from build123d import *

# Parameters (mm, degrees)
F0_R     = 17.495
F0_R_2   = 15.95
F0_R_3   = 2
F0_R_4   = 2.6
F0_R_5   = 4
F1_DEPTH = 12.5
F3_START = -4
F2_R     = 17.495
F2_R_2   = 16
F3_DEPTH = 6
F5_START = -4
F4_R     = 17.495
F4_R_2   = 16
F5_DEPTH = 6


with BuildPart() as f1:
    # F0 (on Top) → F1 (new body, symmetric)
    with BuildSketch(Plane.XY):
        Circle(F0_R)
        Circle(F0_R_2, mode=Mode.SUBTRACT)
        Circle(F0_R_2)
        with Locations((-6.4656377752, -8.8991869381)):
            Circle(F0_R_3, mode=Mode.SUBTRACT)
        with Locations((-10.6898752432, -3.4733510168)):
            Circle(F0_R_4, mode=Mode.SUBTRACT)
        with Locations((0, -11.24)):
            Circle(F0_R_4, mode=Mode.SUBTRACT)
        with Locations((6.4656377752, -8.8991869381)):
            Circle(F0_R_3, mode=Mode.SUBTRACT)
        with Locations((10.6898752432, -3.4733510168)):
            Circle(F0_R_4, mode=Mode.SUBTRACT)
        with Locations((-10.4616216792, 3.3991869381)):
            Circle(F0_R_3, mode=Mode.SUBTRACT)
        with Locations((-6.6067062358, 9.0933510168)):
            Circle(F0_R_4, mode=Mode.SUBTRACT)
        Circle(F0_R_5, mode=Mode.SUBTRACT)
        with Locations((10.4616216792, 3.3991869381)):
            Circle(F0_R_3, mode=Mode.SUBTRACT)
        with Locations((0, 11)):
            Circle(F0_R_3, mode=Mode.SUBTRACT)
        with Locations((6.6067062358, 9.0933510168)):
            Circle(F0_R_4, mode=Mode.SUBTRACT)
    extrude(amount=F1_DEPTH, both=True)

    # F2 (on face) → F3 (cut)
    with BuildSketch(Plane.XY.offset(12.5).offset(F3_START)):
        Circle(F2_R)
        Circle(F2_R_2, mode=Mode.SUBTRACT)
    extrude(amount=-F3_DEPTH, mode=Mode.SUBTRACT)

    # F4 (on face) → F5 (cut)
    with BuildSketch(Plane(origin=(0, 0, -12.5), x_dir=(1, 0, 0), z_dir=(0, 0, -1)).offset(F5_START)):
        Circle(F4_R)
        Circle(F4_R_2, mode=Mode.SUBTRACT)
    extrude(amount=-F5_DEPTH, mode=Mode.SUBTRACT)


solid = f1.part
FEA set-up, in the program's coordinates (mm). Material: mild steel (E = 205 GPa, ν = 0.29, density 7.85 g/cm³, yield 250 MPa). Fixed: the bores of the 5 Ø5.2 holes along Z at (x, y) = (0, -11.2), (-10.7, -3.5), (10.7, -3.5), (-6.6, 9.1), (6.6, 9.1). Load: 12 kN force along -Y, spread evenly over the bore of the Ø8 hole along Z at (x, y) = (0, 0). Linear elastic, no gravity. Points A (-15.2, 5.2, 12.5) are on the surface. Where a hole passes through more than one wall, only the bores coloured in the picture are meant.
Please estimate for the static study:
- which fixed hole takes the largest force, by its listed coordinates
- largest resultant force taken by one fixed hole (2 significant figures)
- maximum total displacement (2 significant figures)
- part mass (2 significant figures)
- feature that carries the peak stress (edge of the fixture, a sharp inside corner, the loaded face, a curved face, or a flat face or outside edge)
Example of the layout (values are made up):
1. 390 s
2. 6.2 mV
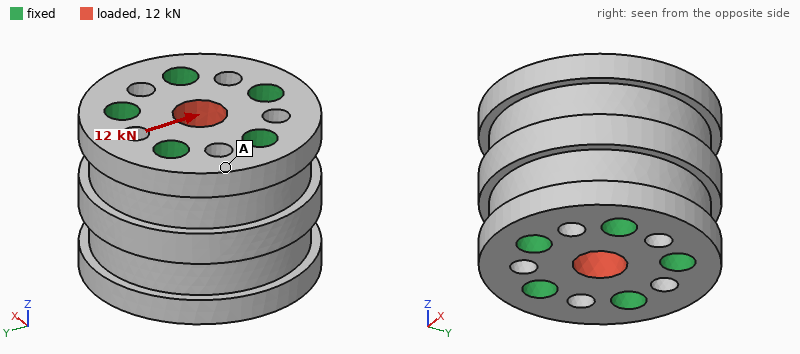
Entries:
1. (0, -11.2)
2. 3.8 kN
3. 0.67 µm
4. 130 g
5. the loaded face
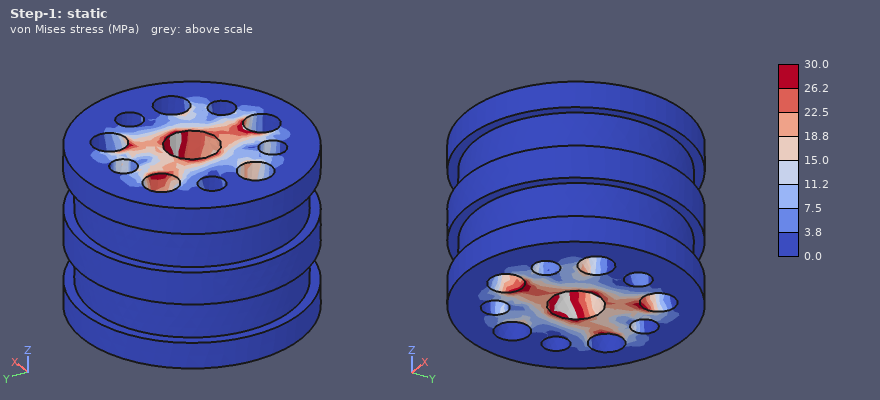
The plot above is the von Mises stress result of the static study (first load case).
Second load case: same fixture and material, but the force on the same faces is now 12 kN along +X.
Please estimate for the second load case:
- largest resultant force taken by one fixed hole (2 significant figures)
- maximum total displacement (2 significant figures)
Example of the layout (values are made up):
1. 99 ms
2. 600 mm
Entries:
1. 3.7 kN
2. 0.66 µm
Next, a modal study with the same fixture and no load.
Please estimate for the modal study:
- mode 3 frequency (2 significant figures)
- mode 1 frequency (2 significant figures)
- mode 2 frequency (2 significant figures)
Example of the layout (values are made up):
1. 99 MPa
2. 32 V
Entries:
1. 110 kHz
2. 110 kHz
3. 110 kHz
